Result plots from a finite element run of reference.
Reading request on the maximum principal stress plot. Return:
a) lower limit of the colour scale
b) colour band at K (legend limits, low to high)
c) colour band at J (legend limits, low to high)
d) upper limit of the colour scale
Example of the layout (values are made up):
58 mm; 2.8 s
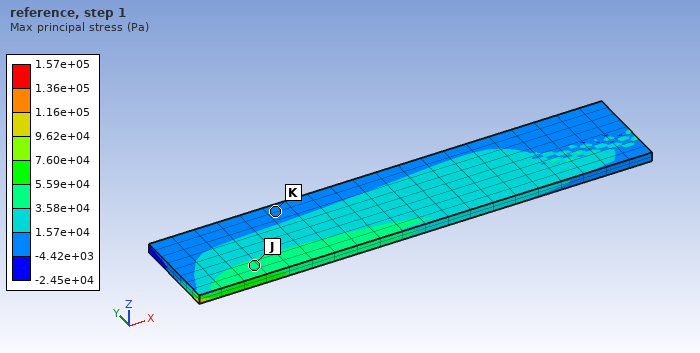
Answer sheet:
-2.45e+04 Pa; -4.42e+03 to 1.57e+04 Pa; 3.58e+04 to 5.59e+04 Pa; 1.57e+05 Pa
